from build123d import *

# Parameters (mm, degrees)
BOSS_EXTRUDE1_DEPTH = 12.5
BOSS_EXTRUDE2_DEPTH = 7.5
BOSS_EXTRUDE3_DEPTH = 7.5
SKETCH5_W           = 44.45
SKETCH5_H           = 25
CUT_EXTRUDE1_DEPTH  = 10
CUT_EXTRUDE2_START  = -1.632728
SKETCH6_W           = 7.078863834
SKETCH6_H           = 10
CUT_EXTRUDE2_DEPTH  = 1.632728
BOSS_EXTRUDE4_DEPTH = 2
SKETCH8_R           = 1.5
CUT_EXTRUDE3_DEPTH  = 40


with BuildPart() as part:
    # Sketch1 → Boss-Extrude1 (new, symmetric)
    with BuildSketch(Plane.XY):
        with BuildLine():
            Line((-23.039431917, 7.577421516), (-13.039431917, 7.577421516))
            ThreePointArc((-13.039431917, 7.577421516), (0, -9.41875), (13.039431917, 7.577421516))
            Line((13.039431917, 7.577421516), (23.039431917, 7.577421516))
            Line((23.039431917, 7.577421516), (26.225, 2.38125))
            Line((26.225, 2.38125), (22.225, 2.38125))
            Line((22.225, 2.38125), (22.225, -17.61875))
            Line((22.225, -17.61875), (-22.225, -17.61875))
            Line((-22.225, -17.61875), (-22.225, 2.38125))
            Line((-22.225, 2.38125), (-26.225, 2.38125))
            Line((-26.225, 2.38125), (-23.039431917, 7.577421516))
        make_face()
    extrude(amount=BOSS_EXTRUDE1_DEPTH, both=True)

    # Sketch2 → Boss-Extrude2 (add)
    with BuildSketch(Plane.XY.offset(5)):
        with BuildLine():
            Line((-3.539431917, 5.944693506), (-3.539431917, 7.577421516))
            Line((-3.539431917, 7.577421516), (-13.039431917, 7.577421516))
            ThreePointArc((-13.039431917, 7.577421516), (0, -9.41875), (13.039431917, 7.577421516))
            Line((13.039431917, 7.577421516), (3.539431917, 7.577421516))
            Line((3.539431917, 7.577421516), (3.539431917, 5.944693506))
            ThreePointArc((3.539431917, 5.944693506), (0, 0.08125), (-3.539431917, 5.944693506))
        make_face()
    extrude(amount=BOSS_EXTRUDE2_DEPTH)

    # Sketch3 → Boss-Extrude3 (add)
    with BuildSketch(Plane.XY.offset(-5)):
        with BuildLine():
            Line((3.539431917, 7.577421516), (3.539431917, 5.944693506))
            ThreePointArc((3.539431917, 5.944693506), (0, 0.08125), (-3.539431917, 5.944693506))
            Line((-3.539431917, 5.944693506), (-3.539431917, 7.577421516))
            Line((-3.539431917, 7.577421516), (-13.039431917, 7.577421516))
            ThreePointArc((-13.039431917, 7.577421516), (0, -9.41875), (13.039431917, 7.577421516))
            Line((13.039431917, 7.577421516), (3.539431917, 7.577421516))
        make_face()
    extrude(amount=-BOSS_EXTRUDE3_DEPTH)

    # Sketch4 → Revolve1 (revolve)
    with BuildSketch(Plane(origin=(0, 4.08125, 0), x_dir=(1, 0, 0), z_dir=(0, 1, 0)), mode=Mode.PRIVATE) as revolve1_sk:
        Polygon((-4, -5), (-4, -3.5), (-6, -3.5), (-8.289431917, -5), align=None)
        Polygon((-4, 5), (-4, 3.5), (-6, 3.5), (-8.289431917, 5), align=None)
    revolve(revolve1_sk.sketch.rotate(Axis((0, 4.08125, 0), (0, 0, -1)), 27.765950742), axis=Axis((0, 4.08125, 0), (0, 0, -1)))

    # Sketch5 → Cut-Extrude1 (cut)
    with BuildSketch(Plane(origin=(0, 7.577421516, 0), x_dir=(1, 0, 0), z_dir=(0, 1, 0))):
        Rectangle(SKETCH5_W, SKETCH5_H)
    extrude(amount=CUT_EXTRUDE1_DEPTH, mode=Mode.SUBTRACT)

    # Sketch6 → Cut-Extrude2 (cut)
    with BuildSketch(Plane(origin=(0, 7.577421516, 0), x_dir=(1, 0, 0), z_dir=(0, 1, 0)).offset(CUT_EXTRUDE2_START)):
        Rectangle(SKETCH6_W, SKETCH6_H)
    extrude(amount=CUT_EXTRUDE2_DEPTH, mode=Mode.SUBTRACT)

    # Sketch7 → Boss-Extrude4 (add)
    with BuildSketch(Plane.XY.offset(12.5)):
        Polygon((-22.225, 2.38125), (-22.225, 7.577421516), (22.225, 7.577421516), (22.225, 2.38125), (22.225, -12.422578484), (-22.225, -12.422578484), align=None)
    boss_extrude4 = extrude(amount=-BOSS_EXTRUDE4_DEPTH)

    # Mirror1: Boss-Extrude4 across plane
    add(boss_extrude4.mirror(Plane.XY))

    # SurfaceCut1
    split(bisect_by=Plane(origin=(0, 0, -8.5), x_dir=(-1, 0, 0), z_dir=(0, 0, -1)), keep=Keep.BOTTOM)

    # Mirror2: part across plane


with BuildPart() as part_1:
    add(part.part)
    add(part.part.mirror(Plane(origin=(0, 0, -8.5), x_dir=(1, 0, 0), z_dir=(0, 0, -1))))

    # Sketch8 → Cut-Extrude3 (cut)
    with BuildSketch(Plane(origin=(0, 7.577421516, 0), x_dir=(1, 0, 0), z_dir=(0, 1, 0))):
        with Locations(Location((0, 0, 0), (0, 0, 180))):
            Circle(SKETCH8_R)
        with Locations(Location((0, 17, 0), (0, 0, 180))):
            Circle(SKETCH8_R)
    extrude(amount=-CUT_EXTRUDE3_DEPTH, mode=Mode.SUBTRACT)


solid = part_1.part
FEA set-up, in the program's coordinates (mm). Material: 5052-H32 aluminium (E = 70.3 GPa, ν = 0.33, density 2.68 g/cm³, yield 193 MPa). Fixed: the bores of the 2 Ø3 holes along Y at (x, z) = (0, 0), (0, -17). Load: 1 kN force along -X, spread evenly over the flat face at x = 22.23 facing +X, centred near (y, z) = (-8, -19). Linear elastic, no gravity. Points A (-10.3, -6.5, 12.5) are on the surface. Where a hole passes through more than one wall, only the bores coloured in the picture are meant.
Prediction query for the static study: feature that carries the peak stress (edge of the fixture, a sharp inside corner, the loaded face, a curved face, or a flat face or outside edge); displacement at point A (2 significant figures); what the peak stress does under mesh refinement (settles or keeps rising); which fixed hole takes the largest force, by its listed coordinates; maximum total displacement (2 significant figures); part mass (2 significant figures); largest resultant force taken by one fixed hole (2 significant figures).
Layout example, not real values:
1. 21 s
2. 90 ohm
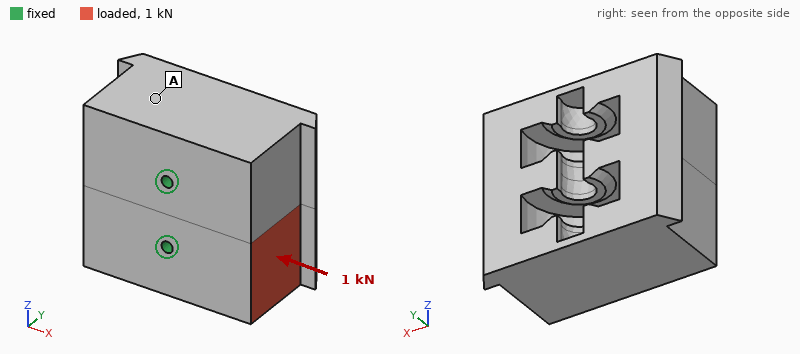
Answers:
1. edge of the fixture
2. 2.2 µm
3. keeps rising
4. (0, -17)
5. 9.8 µm
6. 110 g
7. 1.1 kN
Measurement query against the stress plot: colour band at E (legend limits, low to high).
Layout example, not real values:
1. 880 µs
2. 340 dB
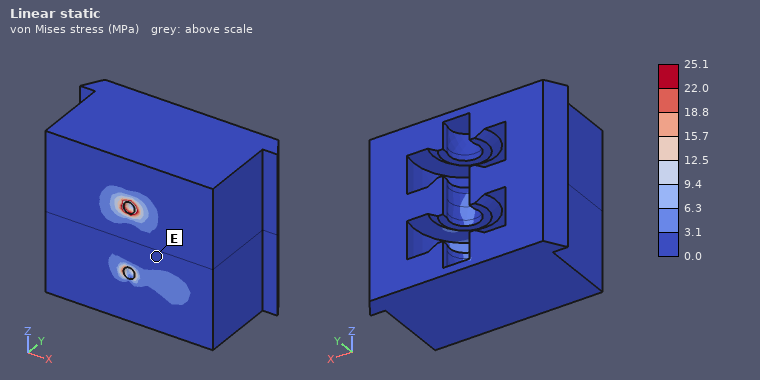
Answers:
1. 0.0 to 3.1 MPa
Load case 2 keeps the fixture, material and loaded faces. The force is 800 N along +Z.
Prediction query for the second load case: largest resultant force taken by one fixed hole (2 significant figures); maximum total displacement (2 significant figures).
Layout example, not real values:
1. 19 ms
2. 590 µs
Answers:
1. 1.1 kN
2. 6.6 µm
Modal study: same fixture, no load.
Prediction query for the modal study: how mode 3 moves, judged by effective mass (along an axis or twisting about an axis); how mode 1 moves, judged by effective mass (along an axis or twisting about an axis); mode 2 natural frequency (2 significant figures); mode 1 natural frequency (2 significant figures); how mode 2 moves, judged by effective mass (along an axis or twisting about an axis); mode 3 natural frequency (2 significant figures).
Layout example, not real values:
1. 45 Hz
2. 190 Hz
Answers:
1. twisting about Y
2. along X
3. 8500 Hz
4. 4400 Hz
5. along Z
6. 9700 Hz
